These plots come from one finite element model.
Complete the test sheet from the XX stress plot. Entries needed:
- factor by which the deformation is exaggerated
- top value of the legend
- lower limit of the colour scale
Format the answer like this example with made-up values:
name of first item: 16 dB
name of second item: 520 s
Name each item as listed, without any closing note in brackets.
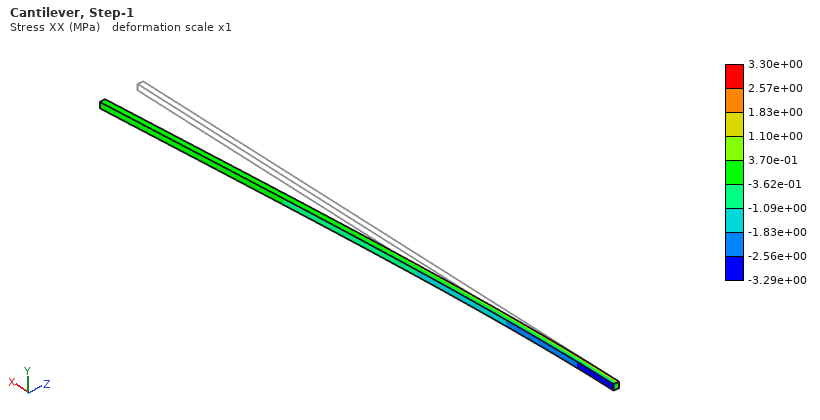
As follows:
factor by which the deformation is exaggerated: 1
top value of the legend: 3.30e+00 MPa
lower limit of the colour scale: -3.29e+00 MPa
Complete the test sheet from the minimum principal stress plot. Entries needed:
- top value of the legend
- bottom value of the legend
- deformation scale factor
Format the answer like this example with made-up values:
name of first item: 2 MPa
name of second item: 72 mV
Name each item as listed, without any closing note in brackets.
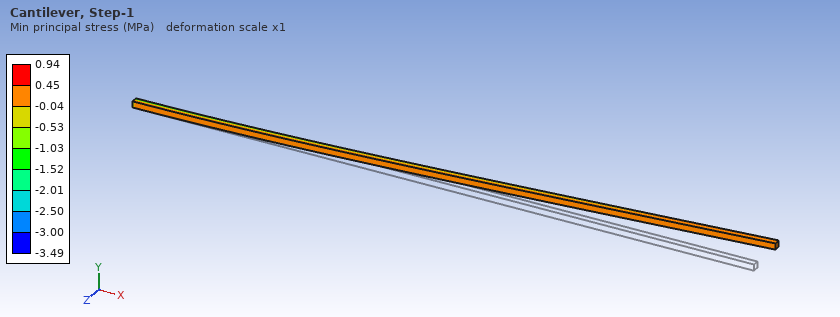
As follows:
top value of the legend: 0.94 MPa
bottom value of the legend: -3.49 MPa
deformation scale factor: 1
